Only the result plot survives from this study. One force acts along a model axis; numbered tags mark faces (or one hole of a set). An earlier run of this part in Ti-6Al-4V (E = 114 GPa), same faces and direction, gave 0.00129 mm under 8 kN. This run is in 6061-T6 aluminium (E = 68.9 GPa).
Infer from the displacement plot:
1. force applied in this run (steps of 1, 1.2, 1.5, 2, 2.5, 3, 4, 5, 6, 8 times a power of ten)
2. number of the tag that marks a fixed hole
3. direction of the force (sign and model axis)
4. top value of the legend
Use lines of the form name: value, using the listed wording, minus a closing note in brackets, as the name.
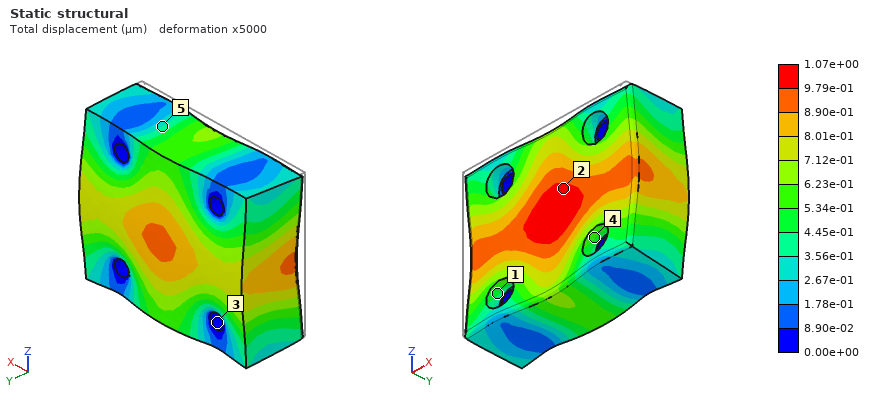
force applied in this run: 4 kN
number of the tag that marks a fixed hole: 3
direction of the force: +Y
top value of the legend: 1.07e+00 µm
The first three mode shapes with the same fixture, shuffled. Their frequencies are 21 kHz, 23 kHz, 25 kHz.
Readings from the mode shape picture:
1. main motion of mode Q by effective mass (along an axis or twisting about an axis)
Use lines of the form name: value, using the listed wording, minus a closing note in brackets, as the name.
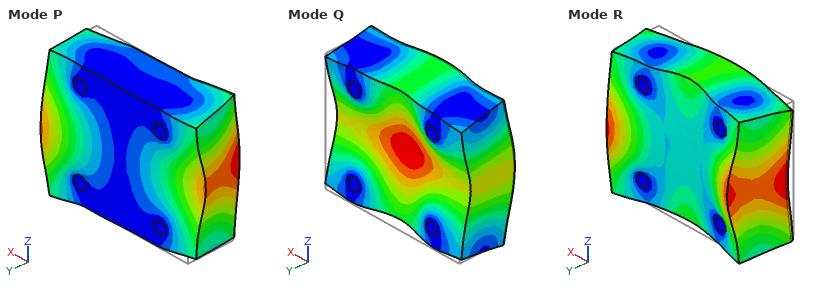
main motion of mode Q by effective mass: along Y
